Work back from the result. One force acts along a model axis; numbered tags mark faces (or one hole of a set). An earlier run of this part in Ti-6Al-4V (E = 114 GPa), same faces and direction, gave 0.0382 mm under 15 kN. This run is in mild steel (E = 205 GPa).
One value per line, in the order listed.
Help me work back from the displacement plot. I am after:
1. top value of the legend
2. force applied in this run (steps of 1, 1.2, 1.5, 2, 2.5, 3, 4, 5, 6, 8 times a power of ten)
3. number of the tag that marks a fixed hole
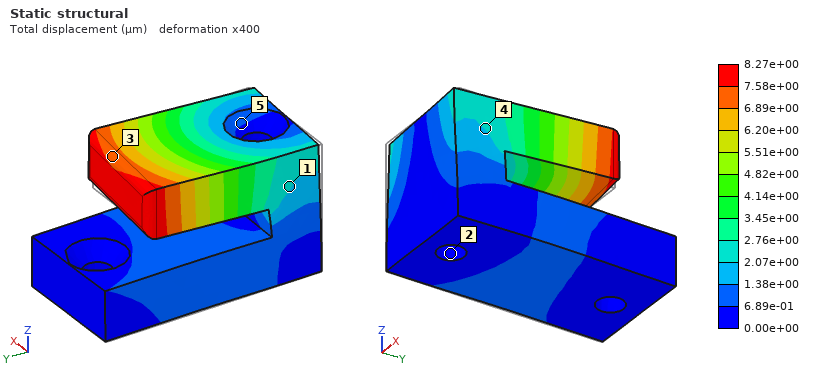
8.27e+00 µm
6 kN
2
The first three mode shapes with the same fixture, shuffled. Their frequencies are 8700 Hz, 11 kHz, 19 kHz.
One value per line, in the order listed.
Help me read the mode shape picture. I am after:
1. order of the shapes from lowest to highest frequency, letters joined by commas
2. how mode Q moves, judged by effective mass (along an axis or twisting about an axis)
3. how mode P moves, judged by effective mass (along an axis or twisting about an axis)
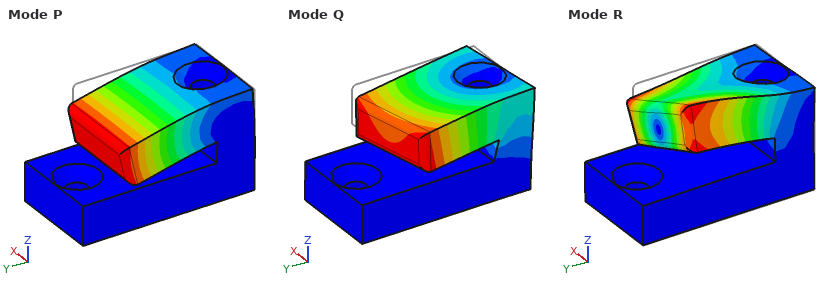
P, Q, R
along X
along Z
